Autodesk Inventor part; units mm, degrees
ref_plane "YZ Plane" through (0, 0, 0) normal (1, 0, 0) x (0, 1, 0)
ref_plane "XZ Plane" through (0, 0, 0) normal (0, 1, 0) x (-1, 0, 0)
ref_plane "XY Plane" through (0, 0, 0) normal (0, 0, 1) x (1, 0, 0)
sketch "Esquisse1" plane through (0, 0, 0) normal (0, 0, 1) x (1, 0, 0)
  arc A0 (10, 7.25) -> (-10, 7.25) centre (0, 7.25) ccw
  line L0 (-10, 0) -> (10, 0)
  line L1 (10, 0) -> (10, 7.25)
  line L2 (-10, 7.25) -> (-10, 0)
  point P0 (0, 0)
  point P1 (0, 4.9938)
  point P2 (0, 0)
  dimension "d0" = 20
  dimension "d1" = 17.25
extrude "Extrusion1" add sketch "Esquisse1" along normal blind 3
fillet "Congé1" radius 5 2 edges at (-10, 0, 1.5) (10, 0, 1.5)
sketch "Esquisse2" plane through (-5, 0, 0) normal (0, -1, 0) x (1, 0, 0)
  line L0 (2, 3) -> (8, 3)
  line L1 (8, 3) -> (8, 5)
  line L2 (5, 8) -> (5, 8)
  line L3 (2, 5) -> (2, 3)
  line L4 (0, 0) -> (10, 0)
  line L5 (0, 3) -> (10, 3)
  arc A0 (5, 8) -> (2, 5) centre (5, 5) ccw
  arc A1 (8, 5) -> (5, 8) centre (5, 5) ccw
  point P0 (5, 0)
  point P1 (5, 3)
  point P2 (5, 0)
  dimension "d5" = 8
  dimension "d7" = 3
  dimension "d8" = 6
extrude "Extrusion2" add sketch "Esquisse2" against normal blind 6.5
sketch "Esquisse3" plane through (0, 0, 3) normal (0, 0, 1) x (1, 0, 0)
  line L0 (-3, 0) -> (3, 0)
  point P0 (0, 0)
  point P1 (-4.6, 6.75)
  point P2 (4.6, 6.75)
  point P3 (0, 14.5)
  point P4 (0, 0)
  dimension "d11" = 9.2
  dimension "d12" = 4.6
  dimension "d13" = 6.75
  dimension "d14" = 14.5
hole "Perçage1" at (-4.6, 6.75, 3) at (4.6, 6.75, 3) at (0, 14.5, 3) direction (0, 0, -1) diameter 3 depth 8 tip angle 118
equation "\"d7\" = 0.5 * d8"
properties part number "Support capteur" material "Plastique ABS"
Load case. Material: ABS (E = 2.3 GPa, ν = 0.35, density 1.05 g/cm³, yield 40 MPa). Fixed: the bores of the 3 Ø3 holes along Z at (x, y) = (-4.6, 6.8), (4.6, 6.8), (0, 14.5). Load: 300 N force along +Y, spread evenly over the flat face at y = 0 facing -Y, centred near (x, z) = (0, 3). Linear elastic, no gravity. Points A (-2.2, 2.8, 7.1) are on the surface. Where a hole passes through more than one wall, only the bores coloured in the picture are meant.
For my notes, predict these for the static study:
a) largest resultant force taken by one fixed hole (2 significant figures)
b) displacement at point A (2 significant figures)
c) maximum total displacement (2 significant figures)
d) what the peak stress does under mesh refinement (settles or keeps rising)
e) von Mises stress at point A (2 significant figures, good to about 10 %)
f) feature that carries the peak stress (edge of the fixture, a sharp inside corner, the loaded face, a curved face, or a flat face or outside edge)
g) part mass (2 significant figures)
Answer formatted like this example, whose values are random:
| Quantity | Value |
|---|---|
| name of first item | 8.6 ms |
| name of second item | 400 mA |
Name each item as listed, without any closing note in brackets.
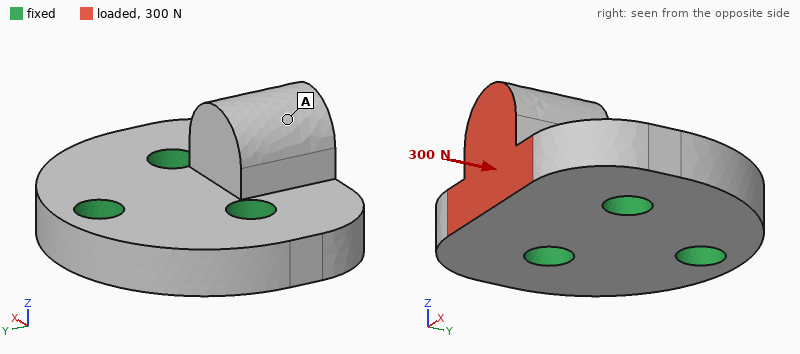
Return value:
| Quantity | Value |
|---|---|
| largest resultant force taken by one fixed hole | 140 N |
| displacement at point A | 0.11 mm |
| maximum total displacement | 0.15 mm |
| what the peak stress does under mesh refinement | keeps rising |
| von Mises stress at point A | 4.3 MPa |
| feature that carries the peak stress | edge of the fixture |
| part mass | 1.0 g |
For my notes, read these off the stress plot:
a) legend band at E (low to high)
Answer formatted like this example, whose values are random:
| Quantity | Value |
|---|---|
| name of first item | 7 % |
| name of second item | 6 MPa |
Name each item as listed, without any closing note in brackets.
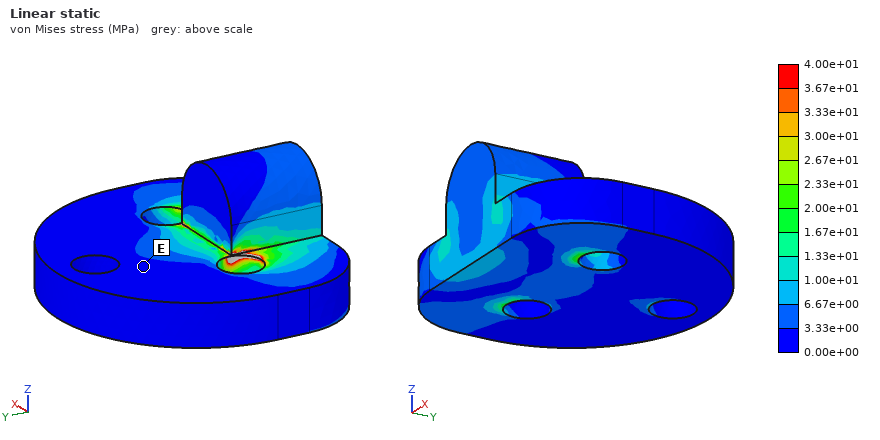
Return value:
| Quantity | Value |
|---|---|
| legend band at E | 0.00e+00 to 3.33e+00 MPa |
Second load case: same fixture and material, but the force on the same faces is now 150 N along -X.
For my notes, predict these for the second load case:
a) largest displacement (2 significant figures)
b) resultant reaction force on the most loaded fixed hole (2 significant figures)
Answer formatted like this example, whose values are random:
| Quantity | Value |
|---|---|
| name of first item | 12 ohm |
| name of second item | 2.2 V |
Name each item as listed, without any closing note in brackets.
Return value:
| Quantity | Value |
|---|---|
| largest displacement | 53 µm |
| resultant reaction force on the most loaded fixed hole | 120 N |
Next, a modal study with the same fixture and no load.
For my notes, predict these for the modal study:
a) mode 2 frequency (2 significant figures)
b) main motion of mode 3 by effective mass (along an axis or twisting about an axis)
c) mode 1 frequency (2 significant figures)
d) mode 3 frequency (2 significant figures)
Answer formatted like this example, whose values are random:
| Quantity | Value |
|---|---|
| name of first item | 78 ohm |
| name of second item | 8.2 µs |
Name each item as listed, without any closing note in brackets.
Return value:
| Quantity | Value |
|---|---|
| mode 2 frequency | 20 kHz |
| main motion of mode 3 by effective mass | twisting about Y |
| mode 1 frequency | 11 kHz |
| mode 3 frequency | 22 kHz |
